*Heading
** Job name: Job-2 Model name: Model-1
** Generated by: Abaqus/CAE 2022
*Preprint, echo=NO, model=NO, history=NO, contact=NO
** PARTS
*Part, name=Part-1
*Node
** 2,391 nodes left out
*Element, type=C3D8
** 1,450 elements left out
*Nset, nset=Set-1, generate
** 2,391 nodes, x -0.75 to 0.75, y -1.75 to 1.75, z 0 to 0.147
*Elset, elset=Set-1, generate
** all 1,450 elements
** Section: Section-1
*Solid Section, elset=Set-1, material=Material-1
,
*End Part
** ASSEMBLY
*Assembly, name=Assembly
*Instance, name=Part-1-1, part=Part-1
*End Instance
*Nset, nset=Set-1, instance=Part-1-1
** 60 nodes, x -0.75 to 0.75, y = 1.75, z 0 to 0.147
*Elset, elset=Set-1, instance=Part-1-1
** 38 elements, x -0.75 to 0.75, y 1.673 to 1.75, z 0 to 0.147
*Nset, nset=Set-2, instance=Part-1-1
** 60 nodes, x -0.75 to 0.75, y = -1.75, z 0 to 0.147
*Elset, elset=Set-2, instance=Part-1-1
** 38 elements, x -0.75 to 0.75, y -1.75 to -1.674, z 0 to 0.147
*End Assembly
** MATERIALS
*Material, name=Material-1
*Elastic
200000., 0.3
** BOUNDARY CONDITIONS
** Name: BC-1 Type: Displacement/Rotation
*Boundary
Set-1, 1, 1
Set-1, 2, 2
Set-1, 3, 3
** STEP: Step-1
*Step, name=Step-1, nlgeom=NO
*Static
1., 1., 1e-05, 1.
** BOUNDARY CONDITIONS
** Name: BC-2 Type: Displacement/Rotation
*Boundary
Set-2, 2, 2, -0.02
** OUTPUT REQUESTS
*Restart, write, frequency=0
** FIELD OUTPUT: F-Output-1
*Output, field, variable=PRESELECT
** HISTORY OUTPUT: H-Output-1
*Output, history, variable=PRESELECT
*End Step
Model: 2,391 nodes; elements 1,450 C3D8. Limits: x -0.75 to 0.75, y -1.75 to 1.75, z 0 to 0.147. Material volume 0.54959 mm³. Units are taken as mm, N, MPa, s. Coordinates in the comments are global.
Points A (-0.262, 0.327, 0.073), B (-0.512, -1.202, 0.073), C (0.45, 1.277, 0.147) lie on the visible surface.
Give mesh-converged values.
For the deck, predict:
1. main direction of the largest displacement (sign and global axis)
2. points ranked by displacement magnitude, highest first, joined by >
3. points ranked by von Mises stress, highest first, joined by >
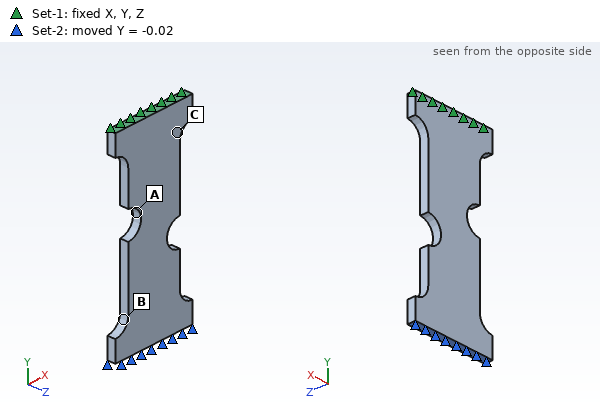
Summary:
-Y
B > A > C
A > B > C
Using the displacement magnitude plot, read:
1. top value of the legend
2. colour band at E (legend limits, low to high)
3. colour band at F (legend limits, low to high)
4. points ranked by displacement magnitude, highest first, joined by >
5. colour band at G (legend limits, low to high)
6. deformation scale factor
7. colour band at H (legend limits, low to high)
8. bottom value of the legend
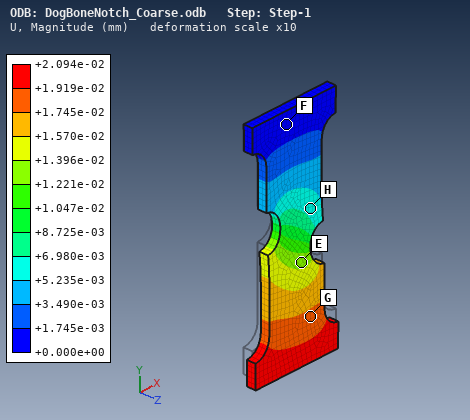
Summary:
+2.094e-02 mm
+1.221e-02 to +1.396e-02 mm
+0.000e+00 to +1.745e-03 mm
G > E > H > F
+1.745e-02 to +1.919e-02 mm
10
+5.235e-03 to +6.980e-03 mm
+0.000e+00 mm
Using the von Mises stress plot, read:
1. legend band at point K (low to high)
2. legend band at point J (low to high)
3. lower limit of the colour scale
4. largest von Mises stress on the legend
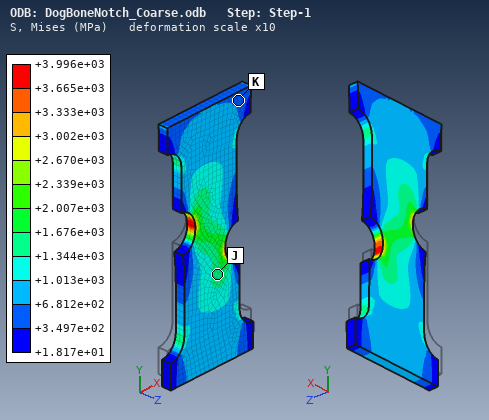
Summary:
+3.497e+02 to +6.812e+02 MPa
+1.344e+03 to +1.676e+03 MPa
+1.817e+01 MPa
+3.996e+03 MPa
